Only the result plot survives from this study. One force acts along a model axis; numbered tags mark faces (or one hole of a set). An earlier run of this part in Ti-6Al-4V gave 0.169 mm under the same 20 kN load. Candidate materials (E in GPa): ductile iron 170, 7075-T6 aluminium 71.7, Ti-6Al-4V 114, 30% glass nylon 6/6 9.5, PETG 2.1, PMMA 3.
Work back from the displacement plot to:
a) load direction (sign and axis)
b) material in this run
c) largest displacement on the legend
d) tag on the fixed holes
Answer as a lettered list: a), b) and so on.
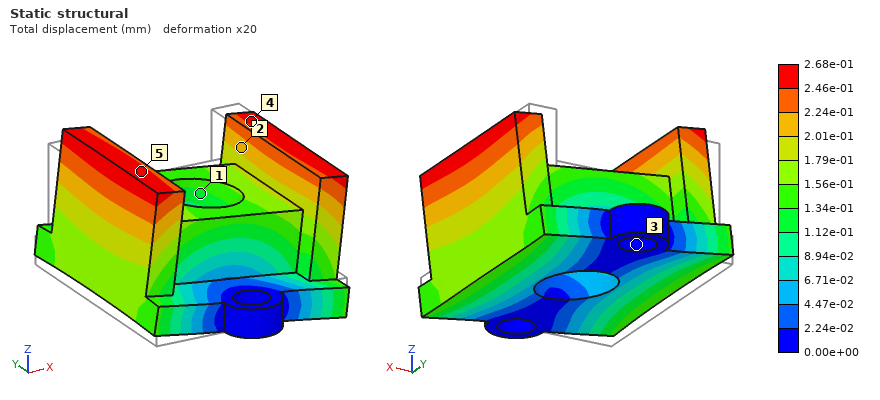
a) +X
b) 7075-T6 aluminium
c) 2.68e-01 mm
d) 3
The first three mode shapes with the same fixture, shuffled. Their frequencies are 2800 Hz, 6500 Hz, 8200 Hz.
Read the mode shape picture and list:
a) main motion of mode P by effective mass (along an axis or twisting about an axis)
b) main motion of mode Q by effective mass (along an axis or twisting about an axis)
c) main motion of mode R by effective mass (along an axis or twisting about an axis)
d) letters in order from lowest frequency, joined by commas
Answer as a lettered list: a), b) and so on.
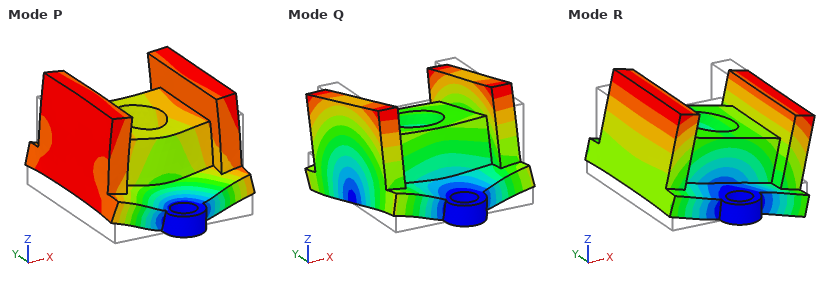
a) along Z
b) along Y
c) along X
d) R, P, Q
